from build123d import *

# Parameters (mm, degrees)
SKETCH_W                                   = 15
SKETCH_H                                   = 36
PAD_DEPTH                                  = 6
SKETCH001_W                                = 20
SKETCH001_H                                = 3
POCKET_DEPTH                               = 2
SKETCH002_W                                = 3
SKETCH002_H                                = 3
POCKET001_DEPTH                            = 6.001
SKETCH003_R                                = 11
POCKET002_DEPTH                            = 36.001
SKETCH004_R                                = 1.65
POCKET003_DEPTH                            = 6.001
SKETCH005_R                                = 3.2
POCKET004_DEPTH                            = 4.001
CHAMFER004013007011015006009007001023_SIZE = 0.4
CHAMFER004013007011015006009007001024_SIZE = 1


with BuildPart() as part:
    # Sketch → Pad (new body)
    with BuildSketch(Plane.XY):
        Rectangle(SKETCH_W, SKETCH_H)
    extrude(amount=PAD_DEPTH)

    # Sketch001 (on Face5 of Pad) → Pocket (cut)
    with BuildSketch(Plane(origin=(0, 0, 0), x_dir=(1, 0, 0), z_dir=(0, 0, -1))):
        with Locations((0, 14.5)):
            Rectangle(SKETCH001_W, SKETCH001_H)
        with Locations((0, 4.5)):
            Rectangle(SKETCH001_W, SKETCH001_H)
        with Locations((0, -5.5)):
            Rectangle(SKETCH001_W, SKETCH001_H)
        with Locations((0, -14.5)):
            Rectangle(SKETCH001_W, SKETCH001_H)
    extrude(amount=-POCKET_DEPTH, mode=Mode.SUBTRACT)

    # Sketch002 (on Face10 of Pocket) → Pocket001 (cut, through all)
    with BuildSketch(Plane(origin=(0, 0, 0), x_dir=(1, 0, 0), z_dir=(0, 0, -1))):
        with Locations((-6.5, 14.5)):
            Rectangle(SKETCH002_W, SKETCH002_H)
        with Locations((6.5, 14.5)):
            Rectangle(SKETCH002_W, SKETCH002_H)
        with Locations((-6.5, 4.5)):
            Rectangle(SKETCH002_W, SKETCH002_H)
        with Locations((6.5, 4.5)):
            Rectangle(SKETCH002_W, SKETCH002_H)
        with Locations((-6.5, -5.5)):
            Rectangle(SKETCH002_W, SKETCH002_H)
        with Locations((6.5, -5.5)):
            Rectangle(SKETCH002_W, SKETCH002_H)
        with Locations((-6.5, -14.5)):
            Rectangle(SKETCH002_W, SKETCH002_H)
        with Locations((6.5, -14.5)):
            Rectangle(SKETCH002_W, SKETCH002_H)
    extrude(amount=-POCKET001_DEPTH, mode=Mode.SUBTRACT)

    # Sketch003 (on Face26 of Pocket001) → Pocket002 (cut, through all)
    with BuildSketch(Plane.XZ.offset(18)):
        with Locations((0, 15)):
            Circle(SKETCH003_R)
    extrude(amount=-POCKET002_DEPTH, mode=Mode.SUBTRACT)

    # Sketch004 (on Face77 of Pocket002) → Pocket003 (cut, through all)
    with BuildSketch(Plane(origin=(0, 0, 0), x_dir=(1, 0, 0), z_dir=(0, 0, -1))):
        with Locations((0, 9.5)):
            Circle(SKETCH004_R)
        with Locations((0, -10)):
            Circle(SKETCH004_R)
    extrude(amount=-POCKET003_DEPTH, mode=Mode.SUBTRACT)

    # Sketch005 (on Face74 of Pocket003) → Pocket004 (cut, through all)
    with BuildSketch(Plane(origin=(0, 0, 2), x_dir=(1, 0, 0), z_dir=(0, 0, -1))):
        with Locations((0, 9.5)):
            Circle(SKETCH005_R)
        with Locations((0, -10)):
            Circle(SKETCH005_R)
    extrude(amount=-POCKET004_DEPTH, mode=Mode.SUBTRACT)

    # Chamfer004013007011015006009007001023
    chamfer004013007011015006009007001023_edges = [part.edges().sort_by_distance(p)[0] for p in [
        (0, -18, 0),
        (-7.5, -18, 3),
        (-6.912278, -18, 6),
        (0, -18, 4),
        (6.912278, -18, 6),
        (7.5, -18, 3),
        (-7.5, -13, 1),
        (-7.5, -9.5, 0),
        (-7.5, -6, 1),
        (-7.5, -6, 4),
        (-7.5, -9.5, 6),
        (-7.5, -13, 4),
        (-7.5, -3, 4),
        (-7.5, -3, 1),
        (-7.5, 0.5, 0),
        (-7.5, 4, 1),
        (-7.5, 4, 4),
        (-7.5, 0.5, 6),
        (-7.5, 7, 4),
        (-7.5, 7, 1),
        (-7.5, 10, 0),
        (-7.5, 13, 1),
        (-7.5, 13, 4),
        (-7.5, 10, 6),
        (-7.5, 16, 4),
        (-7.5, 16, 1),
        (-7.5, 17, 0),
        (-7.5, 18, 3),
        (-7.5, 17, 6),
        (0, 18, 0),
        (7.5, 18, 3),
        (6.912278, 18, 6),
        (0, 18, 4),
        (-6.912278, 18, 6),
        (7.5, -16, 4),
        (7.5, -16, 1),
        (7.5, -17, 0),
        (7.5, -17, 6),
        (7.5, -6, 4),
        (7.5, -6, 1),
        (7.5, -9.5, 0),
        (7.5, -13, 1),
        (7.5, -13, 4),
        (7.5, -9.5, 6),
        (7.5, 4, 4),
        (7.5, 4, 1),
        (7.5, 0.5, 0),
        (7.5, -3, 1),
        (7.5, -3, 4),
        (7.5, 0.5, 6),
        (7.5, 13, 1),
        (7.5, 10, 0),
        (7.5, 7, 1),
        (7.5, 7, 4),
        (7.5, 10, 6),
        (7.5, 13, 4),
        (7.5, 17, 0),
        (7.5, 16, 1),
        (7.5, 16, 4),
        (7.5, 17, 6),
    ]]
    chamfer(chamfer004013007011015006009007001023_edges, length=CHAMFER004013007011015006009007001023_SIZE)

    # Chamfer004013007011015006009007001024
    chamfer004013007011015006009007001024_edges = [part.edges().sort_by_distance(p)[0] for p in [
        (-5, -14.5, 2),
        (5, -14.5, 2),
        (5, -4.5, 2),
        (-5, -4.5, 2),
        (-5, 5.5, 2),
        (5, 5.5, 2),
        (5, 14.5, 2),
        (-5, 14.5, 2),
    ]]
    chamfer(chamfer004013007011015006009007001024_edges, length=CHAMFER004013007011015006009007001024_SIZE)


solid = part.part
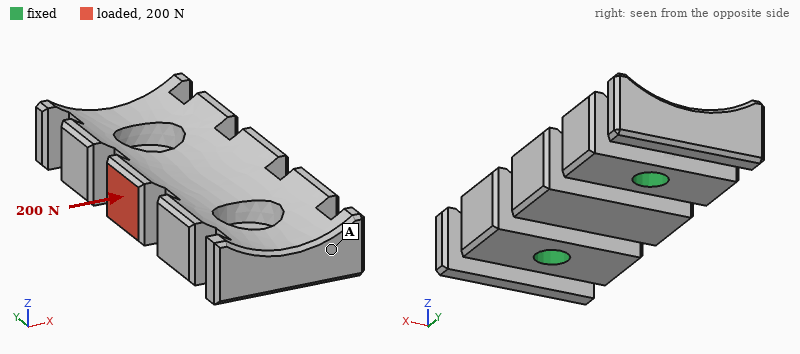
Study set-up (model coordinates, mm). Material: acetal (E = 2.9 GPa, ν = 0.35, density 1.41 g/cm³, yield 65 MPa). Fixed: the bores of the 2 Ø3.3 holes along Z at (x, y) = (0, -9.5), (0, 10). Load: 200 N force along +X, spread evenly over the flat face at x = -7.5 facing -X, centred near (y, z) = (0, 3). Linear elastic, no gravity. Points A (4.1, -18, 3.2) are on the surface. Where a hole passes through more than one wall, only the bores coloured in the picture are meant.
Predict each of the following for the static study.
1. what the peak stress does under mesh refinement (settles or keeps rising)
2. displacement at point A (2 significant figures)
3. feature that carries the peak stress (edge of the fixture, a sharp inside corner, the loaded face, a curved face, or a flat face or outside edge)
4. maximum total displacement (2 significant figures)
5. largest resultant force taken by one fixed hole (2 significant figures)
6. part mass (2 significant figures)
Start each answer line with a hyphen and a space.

- keeps rising
- 0.024 mm
- a sharp inside corner
- 0.14 mm
- 100 N
- 2.6 g
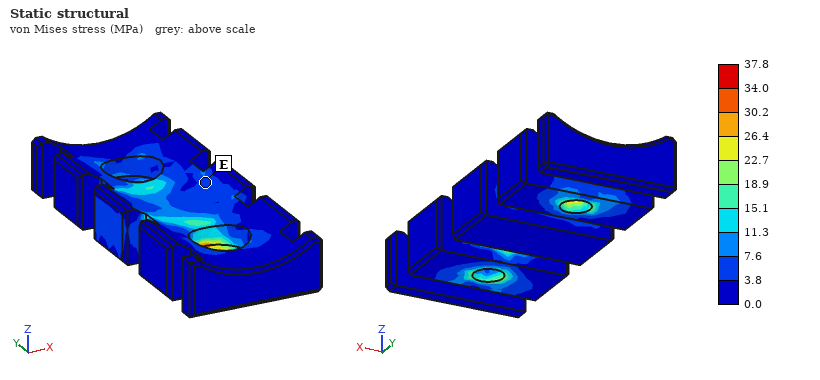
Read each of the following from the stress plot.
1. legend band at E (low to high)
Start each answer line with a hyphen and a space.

- 3.8 to 7.6 MPa
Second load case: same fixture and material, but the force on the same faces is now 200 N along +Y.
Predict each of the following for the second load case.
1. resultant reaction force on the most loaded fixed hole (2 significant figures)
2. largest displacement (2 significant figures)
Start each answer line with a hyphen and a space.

- 130 N
- 0.13 mm
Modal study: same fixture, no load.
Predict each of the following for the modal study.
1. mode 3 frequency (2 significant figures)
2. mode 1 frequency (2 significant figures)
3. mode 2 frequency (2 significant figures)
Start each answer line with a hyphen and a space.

- 5900 Hz
- 4800 Hz
- 5800 Hz
